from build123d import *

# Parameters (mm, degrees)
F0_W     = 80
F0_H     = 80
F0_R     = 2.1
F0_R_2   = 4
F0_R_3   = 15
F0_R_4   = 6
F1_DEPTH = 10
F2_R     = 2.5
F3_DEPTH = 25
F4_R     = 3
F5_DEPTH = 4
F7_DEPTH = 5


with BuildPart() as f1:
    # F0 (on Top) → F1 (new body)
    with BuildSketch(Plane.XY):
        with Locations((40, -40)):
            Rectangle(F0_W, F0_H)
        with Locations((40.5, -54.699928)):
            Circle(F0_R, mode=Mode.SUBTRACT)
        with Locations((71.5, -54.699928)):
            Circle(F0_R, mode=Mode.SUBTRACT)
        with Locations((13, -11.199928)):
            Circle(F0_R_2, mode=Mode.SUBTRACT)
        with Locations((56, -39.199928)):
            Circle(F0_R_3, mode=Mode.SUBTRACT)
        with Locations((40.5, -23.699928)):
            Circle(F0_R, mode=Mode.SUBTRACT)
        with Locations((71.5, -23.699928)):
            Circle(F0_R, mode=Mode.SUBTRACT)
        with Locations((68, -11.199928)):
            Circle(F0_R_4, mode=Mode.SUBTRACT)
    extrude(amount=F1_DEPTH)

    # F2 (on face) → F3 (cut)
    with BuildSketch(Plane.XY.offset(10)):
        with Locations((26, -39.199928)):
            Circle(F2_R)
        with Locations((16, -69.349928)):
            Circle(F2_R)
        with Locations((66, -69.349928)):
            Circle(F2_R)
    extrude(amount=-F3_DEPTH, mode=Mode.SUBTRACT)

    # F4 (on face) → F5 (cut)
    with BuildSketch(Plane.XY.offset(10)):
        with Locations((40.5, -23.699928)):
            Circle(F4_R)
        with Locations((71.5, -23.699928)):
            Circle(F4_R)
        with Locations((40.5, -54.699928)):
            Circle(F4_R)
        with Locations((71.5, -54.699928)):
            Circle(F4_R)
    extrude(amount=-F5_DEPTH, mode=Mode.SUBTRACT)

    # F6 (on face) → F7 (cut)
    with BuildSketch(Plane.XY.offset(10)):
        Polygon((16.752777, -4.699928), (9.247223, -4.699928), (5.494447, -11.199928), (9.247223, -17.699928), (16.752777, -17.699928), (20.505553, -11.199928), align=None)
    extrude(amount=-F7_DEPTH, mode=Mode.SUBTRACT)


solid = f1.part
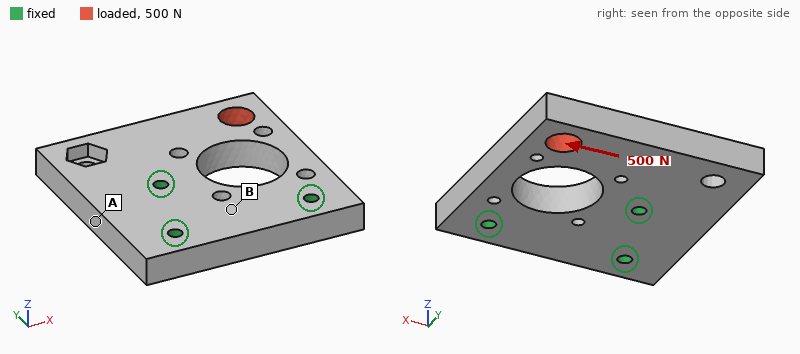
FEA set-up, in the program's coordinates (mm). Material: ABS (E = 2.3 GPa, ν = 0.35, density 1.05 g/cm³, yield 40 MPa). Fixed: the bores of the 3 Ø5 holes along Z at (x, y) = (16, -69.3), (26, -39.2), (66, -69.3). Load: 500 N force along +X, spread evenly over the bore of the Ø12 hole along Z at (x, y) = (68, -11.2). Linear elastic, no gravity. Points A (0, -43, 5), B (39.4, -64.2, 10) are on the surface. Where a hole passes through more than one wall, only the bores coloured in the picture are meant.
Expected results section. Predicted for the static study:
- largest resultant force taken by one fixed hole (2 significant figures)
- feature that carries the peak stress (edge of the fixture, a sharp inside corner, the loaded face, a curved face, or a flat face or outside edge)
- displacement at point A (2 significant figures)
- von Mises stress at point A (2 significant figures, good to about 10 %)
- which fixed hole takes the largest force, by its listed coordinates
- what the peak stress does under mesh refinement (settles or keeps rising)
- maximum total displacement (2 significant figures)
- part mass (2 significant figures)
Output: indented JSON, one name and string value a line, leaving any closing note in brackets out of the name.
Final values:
{
  "largest resultant force taken by one fixed hole": "580 N",
  "feature that carries the peak stress": "edge of the fixture",
  "displacement at point A": "0.028 mm",
  "von Mises stress at point A": "2.4 MPa",
  "which fixed hole takes the largest force, by its listed coordinates": "(26, -39.2)",
  "what the peak stress does under mesh refinement": "keeps rising",
  "maximum total displacement": "0.14 mm",
  "part mass": "56 g"
}
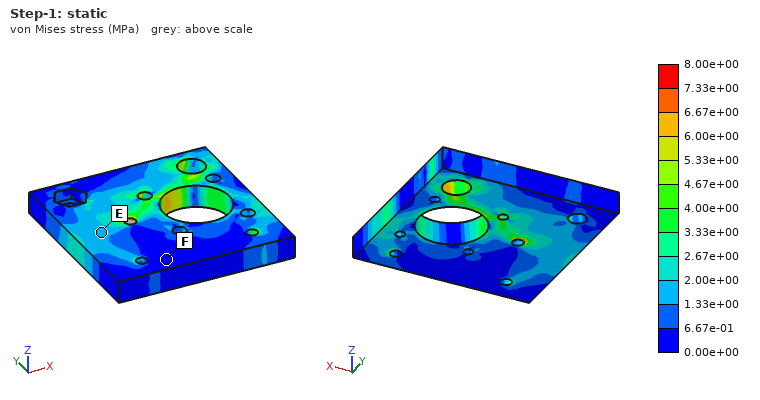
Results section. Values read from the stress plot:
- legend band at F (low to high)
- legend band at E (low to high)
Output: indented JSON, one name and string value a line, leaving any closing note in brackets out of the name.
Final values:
{
  "legend band at F": "0.00e+00 to 6.67e-01 MPa",
  "legend band at E": "1.33e+00 to 2.00e+00 MPa"
}
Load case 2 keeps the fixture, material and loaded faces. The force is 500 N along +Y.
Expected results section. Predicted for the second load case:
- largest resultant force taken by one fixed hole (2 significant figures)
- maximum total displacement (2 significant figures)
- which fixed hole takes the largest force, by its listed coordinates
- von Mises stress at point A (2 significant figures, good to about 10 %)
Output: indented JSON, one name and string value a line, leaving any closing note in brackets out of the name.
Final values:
{
  "largest resultant force taken by one fixed hole": "400 N",
  "maximum total displacement": "0.13 mm",
  "which fixed hole takes the largest force, by its listed coordinates": "(66, -69.3)",
  "von Mises stress at point A": "1.2 MPa"
}
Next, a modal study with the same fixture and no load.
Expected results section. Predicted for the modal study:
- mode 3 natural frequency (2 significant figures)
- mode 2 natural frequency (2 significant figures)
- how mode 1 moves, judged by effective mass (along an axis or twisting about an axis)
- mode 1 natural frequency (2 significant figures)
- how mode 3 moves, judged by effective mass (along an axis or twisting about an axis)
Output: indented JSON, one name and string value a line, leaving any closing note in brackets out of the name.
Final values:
{
  "mode 3 natural frequency": "2400 Hz",
  "mode 2 natural frequency": "1400 Hz",
  "how mode 1 moves, judged by effective mass": "along Z",
  "mode 1 natural frequency": "800 Hz",
  "how mode 3 moves, judged by effective mass": "along X"
}
